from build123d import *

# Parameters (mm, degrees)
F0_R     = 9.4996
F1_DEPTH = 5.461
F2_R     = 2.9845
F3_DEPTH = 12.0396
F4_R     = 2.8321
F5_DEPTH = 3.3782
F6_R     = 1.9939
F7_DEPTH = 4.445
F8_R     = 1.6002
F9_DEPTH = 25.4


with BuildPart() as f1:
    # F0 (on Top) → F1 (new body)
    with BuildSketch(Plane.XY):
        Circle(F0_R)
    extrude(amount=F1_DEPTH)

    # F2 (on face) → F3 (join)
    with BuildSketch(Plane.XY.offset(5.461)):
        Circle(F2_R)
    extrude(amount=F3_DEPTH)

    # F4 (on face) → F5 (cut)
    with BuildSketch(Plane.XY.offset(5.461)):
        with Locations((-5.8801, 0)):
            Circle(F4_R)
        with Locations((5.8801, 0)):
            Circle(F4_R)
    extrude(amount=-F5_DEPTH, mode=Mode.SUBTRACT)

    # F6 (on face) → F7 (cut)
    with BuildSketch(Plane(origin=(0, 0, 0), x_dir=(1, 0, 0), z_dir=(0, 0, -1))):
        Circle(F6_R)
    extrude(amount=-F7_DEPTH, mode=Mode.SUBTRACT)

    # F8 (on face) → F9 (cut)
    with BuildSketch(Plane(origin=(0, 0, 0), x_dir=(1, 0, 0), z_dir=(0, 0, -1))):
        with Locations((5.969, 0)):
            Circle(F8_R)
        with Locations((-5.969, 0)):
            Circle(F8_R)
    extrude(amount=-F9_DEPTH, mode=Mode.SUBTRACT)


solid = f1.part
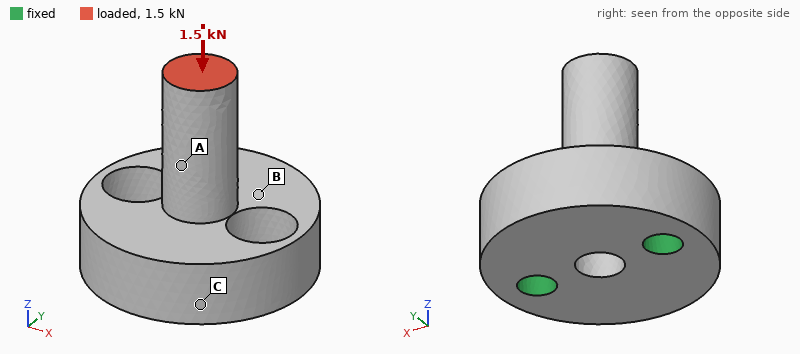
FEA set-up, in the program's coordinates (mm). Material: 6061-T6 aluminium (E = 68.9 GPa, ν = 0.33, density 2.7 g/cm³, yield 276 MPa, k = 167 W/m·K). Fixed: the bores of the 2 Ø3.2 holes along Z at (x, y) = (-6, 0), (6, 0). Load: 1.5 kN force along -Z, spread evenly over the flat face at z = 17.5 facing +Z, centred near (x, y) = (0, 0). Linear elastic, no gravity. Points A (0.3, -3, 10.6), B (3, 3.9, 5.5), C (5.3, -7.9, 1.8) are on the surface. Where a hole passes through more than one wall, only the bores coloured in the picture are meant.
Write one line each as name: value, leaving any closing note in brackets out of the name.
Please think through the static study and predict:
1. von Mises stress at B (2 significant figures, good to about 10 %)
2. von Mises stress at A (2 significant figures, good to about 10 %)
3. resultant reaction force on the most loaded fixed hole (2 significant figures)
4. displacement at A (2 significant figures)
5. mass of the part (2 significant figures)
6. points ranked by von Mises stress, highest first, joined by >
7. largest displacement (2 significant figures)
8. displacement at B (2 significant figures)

von Mises stress at B: 29 MPa
von Mises stress at A: 54 MPa
resultant reaction force on the most loaded fixed hole: 780 N
displacement at A: 12 µm
mass of the part: 4.4 g
points ranked by von Mises stress, highest first, joined by >: A > B > C
largest displacement: 17 µm
displacement at B: 5.4 µm
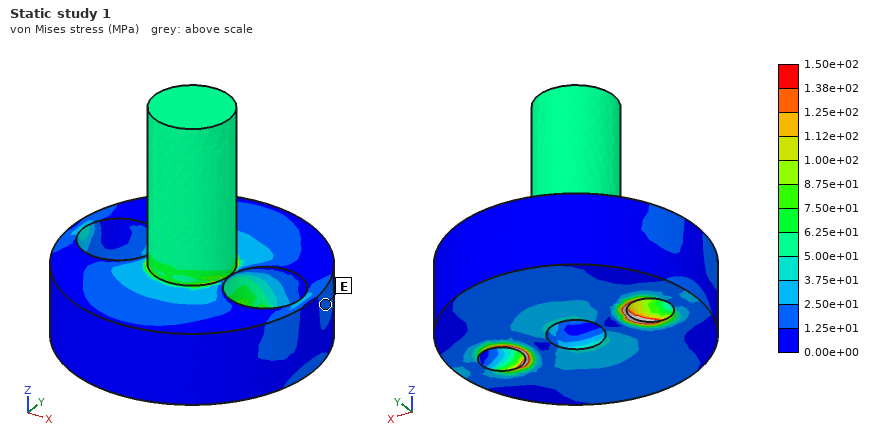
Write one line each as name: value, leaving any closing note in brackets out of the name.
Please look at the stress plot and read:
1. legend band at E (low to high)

legend band at E: 1.25e+01 to 2.50e+01 MPa
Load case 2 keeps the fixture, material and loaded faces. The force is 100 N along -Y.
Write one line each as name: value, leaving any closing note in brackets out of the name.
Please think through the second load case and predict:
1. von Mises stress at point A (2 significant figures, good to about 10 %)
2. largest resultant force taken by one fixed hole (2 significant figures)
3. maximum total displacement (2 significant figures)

von Mises stress at point A: 33 MPa
largest resultant force taken by one fixed hole: 50 N
maximum total displacement: 37 µm
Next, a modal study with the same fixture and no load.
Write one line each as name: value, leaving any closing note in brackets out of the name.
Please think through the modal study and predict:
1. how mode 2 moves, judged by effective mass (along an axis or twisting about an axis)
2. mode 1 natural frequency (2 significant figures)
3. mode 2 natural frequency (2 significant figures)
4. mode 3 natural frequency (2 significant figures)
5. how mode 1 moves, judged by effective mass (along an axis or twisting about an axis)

how mode 2 moves, judged by effective mass: along X
mode 1 natural frequency: 13 kHz
mode 2 natural frequency: 18 kHz
mode 3 natural frequency: 30 kHz
how mode 1 moves, judged by effective mass: along Y
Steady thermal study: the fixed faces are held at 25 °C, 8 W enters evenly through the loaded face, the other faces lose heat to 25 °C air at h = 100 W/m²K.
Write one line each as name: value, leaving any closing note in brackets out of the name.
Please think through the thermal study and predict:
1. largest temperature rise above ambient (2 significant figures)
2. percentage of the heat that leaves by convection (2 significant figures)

largest temperature rise above ambient: 26 K
percentage of the heat that leaves by convection: 7.0 %
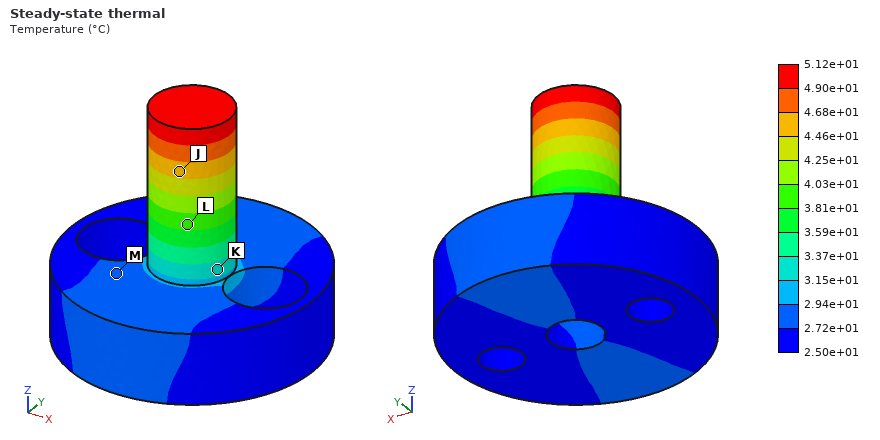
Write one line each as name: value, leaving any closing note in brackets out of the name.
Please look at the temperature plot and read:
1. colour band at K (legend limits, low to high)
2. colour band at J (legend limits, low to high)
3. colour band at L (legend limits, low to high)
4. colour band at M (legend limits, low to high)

colour band at K: 3.15e+01 to 3.37e+01 °C
colour band at J: 4.46e+01 to 4.68e+01 °C
colour band at L: 3.81e+01 to 4.03e+01 °C
colour band at M: 2.72e+01 to 2.94e+01 °C
